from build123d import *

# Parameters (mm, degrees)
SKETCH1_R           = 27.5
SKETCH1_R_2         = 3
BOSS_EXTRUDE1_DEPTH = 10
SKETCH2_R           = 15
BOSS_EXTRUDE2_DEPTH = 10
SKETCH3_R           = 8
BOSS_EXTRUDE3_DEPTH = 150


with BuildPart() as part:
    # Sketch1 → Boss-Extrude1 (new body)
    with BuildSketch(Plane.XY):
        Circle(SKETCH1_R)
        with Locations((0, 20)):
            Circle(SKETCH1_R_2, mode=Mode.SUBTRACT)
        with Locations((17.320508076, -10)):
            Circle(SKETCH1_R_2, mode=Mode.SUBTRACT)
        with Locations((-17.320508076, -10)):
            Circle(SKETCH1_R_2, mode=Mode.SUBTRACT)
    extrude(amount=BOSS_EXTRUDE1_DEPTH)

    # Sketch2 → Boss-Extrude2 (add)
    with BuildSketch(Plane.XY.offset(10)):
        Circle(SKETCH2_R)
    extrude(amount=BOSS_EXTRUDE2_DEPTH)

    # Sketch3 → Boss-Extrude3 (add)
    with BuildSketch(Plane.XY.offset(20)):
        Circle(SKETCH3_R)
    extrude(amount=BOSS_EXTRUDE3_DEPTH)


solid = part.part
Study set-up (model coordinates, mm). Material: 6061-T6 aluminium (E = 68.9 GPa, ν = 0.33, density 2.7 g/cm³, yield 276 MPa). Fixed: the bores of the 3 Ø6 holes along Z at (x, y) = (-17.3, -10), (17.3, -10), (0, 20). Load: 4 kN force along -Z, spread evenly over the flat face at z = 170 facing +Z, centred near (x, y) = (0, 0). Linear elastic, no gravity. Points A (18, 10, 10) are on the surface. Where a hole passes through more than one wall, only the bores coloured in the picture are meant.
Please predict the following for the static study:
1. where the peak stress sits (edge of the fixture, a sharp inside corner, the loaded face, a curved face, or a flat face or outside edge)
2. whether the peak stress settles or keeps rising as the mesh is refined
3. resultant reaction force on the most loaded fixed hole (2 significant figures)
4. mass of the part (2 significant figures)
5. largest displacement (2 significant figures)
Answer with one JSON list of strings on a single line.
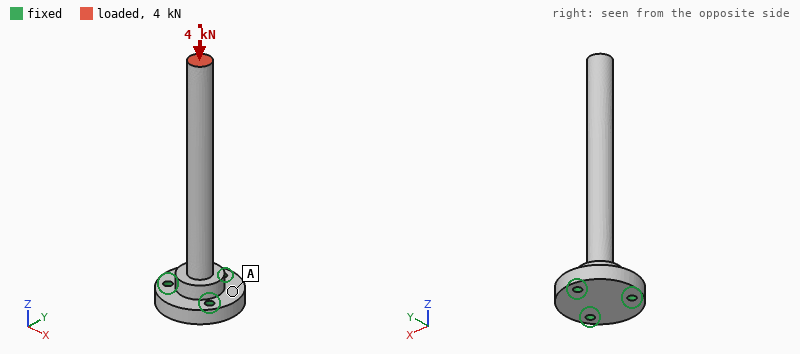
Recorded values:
["edge of the fixture", "keeps rising", "1.4 kN", "160 g", "48 µm"]
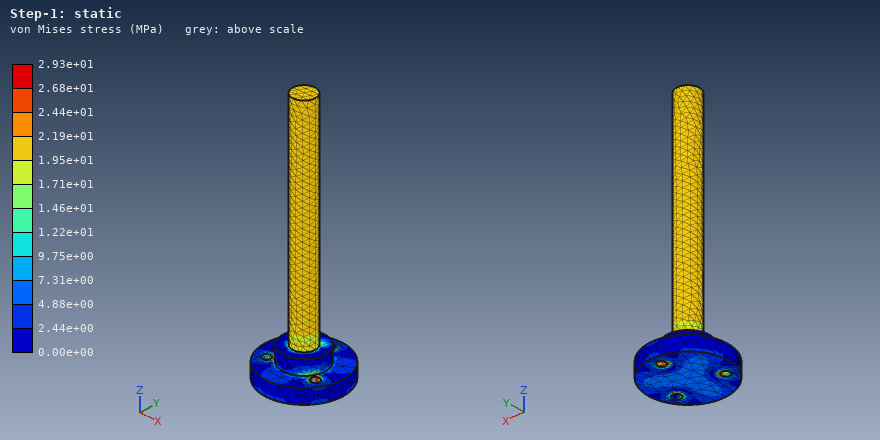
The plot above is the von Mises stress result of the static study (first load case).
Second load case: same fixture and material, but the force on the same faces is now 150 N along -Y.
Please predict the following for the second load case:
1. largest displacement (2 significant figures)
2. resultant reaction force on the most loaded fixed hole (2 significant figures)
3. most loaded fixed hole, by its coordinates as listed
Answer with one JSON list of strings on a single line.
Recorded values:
["0.84 mm", "800 N", "(0, 20)"]
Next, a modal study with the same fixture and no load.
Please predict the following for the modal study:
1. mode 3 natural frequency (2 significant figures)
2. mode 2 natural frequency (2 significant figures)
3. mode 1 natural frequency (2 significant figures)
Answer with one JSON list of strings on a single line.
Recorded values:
["2800 Hz", "470 Hz", "470 Hz"]
